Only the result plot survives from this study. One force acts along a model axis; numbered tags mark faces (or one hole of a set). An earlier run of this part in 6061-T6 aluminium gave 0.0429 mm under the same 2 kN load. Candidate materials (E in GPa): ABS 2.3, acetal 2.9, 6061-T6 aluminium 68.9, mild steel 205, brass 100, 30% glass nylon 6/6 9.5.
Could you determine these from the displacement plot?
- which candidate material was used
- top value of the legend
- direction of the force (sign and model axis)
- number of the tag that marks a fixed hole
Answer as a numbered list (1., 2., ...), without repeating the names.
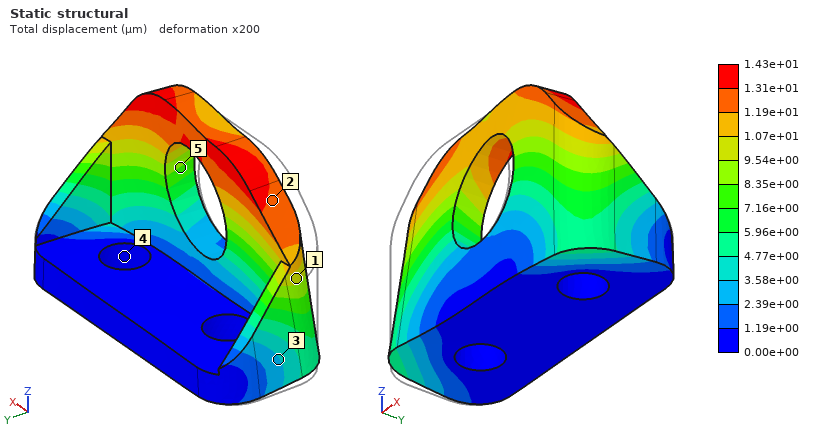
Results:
1. mild steel
2. 1.43e+01 µm
3. +X
4. 4
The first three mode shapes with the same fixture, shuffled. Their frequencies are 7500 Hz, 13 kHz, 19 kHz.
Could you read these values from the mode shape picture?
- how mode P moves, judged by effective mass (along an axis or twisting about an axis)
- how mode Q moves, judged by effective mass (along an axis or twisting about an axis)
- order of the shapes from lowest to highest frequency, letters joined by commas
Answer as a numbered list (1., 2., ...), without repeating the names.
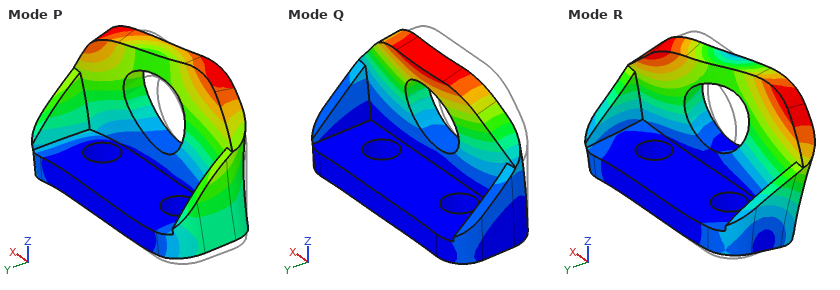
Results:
1. along X
2. along Y
3. Q, R, P
